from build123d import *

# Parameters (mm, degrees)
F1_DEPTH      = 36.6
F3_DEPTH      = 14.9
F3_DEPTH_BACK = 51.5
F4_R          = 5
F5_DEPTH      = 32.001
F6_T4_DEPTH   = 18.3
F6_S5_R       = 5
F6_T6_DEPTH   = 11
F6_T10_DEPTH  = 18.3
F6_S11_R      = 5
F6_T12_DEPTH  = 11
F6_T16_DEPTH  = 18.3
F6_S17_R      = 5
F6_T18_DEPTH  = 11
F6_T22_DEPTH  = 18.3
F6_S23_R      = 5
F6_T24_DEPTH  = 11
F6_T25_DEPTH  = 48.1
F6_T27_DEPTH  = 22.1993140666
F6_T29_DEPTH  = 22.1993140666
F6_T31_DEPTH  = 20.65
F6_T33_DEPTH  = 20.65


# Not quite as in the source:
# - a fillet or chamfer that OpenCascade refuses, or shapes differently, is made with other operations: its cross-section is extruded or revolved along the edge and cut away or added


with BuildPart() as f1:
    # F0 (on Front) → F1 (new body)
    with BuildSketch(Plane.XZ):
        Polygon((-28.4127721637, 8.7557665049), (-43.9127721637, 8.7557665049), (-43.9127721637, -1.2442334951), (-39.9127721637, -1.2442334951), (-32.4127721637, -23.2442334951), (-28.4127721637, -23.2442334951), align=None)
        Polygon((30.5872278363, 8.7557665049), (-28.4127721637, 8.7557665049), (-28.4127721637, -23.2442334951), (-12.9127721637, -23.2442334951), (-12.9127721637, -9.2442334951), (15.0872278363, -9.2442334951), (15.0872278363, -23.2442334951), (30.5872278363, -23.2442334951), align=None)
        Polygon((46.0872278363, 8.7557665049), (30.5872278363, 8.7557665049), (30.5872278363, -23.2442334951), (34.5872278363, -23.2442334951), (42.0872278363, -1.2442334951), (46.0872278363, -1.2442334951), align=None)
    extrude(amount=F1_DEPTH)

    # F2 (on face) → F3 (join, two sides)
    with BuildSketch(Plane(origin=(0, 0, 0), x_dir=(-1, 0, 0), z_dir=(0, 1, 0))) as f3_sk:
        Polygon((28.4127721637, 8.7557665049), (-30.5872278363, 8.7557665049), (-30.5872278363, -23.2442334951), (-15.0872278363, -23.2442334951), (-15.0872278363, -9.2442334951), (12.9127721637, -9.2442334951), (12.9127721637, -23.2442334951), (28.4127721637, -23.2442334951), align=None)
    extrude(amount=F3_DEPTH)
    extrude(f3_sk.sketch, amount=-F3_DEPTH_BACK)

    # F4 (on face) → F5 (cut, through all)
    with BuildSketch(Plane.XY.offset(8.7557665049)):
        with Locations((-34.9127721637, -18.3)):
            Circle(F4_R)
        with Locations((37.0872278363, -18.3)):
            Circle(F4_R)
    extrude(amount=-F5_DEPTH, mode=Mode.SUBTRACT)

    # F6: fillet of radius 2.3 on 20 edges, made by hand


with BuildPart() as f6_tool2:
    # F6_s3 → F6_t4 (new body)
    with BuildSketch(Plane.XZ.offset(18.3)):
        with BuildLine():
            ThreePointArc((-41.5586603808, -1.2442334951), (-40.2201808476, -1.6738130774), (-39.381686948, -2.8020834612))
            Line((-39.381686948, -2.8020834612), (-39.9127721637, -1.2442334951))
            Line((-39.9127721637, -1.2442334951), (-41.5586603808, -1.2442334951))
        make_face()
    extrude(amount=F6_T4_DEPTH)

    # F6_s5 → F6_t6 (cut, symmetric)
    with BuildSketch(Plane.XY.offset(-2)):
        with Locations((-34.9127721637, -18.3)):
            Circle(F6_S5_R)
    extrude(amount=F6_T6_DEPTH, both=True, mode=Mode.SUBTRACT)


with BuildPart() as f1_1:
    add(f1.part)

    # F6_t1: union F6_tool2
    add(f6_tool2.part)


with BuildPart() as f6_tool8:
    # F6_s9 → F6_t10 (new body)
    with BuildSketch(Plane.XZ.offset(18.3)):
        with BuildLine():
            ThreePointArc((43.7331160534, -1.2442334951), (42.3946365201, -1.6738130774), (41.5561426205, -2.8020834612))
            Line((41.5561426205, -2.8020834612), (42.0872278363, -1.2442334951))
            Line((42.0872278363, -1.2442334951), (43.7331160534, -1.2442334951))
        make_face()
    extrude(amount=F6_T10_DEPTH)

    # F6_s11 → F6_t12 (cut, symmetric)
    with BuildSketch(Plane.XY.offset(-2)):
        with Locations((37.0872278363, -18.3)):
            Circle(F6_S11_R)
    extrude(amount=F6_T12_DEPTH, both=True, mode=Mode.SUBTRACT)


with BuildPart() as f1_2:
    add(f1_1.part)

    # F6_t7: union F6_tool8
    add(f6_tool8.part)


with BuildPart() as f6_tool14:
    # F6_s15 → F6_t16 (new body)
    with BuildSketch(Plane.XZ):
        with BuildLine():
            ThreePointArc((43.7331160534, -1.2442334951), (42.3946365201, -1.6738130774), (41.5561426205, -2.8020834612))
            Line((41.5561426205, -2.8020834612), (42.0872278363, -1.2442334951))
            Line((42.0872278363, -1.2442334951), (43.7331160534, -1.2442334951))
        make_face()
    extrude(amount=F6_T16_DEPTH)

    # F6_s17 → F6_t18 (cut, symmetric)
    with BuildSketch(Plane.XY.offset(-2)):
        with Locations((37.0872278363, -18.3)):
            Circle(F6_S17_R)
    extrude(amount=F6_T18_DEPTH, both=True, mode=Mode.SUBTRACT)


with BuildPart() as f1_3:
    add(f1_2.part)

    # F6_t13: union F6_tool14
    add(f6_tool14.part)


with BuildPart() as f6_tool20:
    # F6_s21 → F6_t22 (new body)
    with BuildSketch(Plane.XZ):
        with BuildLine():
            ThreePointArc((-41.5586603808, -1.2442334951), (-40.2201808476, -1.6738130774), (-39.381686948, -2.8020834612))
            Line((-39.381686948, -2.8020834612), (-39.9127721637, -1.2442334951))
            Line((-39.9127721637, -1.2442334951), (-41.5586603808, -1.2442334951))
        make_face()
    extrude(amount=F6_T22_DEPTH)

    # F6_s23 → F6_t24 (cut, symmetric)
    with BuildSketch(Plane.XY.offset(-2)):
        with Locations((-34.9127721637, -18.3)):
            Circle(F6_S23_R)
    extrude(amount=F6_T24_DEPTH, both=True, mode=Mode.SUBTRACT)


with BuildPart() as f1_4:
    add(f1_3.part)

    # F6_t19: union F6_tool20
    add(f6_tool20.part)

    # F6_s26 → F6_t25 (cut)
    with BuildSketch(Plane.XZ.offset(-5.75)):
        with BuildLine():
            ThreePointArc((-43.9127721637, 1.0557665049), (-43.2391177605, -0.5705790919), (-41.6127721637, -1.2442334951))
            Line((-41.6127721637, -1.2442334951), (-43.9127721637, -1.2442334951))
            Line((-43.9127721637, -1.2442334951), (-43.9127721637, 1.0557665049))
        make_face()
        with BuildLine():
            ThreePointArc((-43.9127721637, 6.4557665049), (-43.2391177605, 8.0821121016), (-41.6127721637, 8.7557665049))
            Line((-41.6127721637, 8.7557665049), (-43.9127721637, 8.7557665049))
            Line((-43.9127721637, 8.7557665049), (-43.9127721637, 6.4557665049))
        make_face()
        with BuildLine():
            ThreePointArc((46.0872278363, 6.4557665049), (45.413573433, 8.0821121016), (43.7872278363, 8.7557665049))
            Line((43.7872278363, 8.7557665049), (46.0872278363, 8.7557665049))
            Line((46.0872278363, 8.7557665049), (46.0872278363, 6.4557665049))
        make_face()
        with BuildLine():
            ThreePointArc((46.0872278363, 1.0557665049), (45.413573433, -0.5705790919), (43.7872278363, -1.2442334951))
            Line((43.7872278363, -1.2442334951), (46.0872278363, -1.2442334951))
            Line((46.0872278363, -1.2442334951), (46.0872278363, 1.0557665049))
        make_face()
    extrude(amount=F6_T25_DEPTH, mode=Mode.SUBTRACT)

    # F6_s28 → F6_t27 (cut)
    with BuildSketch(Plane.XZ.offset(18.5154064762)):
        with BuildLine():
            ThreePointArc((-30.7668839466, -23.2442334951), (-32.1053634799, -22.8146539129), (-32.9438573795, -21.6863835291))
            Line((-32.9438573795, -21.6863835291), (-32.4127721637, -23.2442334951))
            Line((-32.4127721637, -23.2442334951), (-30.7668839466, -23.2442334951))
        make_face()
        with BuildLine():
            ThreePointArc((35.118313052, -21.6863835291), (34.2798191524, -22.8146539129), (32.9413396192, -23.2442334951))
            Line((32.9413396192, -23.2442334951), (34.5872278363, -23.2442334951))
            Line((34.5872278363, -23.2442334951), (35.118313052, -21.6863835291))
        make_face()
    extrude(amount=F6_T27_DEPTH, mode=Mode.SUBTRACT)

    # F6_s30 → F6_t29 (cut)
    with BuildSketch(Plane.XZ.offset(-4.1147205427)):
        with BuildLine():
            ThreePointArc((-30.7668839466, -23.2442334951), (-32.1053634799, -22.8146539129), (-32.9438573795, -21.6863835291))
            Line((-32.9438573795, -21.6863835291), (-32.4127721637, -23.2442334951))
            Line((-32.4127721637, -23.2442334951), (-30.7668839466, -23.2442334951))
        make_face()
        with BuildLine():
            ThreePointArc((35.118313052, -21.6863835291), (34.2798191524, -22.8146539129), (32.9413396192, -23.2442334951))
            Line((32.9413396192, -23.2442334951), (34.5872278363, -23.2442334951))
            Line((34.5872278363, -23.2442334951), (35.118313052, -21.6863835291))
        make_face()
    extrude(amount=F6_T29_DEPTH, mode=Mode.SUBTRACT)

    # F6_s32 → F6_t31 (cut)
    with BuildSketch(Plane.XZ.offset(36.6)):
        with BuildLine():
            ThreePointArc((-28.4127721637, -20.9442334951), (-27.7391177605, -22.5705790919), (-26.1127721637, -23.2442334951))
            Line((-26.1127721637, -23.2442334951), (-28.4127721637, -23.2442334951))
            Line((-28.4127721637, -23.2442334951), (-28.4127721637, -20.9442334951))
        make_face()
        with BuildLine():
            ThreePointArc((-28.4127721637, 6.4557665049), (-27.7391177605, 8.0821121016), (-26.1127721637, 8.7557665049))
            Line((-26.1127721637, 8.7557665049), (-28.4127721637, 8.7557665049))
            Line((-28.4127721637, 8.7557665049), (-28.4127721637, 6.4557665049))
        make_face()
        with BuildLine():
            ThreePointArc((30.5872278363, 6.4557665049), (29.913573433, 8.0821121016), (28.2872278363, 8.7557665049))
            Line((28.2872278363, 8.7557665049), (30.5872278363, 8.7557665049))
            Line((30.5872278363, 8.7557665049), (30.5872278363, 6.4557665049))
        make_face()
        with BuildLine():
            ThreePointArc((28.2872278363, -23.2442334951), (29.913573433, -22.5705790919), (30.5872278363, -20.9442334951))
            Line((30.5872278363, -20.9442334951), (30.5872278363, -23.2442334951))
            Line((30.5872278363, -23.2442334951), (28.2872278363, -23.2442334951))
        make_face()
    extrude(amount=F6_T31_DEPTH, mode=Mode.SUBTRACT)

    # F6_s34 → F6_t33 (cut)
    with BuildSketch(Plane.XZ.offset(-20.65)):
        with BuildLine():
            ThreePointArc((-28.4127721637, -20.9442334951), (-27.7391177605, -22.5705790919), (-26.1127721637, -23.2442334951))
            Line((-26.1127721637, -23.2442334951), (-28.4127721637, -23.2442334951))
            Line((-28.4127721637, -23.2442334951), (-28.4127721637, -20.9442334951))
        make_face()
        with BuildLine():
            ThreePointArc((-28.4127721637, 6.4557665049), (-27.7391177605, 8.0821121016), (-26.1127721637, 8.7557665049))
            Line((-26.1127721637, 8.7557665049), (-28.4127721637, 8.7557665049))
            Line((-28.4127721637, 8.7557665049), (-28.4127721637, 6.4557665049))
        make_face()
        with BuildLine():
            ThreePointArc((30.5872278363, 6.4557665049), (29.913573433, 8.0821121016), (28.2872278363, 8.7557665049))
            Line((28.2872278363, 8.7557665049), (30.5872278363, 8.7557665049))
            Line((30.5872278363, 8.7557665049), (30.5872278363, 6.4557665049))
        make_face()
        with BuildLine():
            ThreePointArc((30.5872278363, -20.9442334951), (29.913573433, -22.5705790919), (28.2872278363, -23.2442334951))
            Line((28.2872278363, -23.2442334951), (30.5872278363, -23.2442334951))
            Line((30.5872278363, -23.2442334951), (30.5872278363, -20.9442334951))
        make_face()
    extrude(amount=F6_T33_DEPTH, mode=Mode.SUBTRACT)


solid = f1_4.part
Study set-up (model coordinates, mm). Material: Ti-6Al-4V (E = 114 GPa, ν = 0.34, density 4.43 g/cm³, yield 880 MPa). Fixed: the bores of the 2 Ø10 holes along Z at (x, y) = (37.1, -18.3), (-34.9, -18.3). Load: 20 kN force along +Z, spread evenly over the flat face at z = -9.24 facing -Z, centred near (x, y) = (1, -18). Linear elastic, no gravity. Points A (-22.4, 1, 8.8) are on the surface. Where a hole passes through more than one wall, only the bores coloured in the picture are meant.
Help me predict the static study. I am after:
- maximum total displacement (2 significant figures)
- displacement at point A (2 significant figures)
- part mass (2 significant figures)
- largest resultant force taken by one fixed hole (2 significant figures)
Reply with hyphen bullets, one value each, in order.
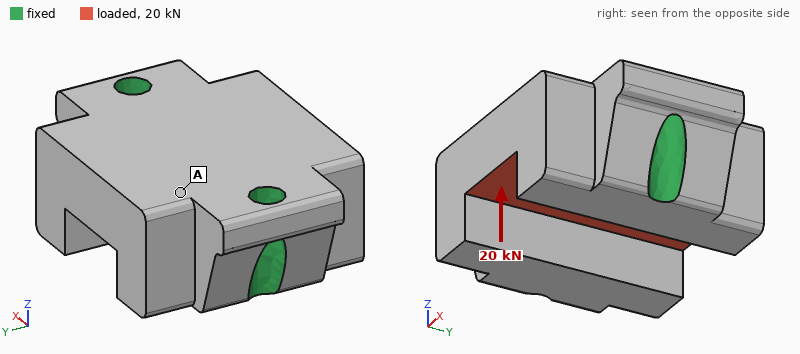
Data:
- 16 µm
- 6.9 µm
- 530 g
- 10 kN
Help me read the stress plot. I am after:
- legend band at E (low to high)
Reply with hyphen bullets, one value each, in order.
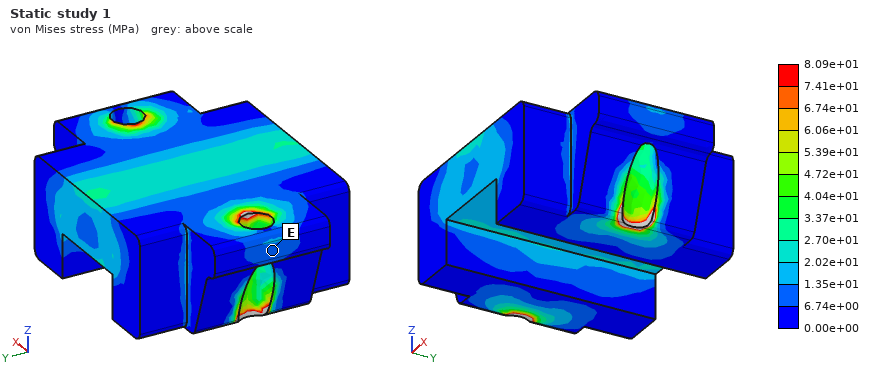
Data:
- 6.74e+00 to 1.35e+01 MPa
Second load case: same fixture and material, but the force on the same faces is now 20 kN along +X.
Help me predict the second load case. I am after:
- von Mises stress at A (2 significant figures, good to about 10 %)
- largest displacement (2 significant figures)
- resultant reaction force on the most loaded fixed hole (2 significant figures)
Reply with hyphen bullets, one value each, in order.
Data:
- 3.1 MPa
- 6.0 µm
- 10 kN
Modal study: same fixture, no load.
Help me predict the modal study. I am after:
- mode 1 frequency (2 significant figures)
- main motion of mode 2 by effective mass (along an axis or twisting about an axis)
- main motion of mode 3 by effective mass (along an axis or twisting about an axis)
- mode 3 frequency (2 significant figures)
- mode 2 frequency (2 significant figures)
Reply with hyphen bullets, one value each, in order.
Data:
- 11 kHz
- along Z
- along Y
- 16 kHz
- 12 kHz
